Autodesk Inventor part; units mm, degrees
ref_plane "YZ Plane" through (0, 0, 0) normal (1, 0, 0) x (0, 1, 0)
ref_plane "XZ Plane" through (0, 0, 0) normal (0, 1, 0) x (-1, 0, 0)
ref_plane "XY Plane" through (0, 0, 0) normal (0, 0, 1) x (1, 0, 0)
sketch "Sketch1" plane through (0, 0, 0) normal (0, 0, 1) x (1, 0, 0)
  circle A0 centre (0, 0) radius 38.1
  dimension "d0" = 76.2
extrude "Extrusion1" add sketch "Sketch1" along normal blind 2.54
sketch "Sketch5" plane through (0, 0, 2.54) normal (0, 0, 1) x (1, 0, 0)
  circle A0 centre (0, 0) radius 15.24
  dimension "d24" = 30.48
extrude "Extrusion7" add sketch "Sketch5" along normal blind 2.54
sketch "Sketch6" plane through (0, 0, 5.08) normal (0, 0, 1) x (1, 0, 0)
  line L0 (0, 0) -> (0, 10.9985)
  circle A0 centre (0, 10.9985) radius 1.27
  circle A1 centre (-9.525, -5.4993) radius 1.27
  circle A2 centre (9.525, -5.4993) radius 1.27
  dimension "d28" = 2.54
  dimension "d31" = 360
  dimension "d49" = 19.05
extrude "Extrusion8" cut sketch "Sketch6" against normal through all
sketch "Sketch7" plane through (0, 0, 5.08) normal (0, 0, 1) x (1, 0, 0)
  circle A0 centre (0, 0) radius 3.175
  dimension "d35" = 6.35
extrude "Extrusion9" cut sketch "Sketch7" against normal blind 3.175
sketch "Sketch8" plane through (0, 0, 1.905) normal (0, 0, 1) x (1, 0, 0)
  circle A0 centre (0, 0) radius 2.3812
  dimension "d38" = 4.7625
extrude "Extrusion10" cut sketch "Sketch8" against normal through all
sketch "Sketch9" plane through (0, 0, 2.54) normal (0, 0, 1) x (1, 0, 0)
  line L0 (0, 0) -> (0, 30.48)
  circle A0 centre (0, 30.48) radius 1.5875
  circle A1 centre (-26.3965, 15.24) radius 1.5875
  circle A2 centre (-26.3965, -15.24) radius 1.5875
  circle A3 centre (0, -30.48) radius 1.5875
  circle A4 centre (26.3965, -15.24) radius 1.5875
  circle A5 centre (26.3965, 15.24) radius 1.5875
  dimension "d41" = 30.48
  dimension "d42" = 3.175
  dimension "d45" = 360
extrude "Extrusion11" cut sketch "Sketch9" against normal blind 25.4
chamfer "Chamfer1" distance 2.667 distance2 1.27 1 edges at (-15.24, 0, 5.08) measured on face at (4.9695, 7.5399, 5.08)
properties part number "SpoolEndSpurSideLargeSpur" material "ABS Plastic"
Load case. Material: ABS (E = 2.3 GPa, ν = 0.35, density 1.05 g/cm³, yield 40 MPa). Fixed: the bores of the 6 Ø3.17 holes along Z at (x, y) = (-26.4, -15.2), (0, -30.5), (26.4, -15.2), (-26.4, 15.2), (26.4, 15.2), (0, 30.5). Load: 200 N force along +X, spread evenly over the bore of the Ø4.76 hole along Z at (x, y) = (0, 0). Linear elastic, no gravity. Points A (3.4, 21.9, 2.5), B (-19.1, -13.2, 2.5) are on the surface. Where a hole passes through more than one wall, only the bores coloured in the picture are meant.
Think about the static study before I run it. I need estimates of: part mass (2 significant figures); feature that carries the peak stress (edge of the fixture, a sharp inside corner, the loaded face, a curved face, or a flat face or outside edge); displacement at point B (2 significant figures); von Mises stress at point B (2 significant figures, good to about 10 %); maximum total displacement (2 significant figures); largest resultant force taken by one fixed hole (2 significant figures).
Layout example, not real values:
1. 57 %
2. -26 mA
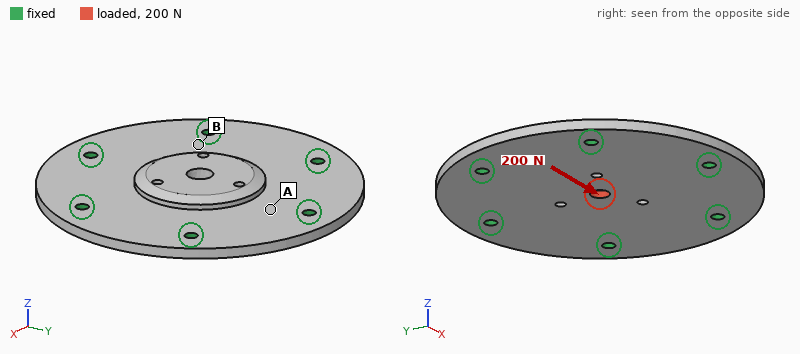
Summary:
1. 14 g
2. a sharp inside corner
3. 5.7 µm
4. 1.4 MPa
5. 29 µm
6. 44 N
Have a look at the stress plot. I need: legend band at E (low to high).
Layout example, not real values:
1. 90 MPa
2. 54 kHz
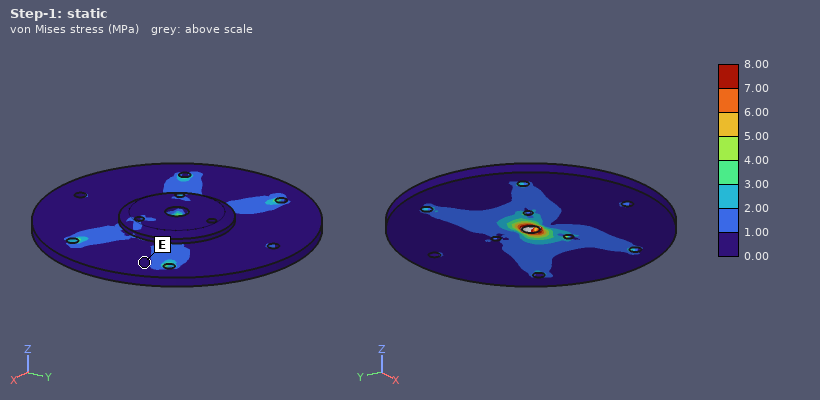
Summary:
1. 0.00 to 1.00 MPa
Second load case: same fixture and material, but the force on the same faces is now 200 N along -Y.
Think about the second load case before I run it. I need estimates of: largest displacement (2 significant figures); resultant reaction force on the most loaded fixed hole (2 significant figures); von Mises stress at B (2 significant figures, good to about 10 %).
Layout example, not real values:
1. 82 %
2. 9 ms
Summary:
1. 29 µm
2. 50 N
3. 0.80 MPa
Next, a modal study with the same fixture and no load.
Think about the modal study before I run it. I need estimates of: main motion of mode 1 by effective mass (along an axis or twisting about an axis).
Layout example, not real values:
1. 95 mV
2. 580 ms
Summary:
1. along Z
